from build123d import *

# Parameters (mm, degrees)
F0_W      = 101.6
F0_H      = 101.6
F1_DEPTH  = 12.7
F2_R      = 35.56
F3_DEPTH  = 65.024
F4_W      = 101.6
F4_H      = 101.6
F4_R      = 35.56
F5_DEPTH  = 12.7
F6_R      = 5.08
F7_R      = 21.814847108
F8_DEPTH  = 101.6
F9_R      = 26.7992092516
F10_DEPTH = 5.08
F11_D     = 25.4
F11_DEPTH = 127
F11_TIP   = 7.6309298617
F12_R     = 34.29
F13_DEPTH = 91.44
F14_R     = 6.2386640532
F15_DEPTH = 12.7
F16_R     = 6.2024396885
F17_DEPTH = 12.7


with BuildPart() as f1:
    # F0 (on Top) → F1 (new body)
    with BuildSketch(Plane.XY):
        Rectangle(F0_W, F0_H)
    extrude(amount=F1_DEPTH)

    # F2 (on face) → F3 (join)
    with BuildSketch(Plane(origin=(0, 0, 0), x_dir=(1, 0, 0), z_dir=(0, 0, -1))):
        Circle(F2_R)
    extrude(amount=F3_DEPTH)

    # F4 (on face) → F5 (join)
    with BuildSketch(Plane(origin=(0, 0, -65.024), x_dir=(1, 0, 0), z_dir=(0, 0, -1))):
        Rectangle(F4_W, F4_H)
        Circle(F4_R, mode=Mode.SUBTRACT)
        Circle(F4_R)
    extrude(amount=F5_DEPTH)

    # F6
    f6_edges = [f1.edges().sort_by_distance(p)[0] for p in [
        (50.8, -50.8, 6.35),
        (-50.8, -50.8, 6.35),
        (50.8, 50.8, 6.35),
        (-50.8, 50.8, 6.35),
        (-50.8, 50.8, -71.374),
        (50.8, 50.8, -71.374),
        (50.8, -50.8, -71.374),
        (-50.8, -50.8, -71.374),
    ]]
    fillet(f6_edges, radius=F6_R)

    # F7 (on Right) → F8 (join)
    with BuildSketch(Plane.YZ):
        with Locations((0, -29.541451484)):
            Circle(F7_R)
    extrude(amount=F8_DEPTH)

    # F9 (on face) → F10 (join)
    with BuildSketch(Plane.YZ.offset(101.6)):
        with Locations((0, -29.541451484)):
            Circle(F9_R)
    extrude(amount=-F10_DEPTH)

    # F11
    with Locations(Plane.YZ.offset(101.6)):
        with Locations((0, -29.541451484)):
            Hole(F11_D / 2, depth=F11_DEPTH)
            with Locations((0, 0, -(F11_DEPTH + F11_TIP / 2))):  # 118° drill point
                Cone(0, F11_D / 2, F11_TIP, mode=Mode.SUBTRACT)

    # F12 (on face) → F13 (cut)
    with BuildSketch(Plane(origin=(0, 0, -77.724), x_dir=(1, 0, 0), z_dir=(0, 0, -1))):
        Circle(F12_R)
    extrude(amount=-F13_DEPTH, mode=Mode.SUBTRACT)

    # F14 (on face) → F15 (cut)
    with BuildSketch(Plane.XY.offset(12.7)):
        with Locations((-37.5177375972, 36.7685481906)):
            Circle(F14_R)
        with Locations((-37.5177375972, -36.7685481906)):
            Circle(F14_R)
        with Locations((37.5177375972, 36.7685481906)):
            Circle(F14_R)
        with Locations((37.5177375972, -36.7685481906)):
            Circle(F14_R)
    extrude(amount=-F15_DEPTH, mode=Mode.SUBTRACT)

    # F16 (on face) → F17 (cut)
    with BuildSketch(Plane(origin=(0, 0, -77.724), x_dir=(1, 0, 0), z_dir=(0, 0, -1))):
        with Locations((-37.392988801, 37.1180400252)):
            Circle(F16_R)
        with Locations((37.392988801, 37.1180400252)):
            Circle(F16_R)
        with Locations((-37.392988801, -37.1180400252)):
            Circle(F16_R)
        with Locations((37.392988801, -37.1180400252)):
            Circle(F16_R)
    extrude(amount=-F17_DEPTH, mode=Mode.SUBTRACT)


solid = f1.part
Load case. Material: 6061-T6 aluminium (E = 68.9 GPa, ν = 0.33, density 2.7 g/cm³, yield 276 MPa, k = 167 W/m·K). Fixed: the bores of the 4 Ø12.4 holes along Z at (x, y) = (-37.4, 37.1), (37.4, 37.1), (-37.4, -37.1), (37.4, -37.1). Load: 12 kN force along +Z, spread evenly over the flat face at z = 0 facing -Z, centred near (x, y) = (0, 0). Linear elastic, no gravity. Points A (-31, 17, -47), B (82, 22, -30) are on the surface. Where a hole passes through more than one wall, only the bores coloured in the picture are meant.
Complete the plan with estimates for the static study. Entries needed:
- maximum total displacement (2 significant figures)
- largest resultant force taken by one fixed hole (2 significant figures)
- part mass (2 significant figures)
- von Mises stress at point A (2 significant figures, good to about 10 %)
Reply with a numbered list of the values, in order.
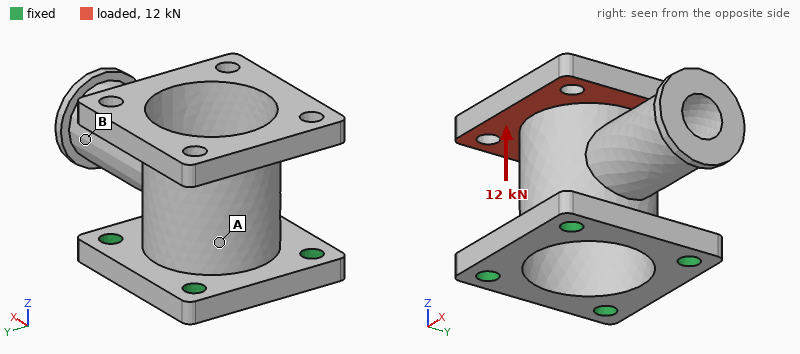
1. 0.19 mm
2. 3.0 kN
3. 660 g
4. 43 MPa
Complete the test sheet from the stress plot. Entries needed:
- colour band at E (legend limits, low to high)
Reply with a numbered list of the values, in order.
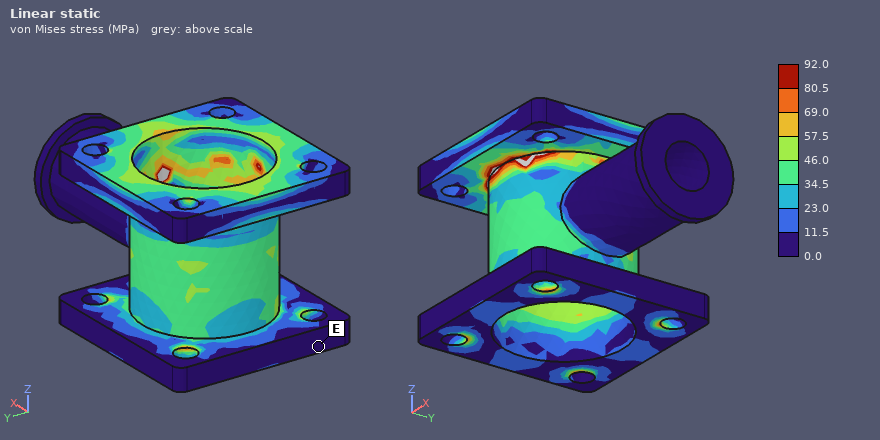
1. 0.0 to 11.5 MPa
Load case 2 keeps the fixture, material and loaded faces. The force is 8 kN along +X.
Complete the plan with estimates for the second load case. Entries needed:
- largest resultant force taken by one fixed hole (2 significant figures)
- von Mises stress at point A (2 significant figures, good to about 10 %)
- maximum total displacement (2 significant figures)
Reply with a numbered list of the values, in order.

1. 5.1 kN
2. 71 MPa
3. 0.40 mm
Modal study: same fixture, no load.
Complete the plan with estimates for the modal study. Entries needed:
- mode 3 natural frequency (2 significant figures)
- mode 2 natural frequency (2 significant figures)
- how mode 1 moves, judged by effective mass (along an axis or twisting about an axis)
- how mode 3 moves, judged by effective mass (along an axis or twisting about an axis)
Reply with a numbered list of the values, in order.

1. 1600 Hz
2. 1100 Hz
3. along Y
4. along Y
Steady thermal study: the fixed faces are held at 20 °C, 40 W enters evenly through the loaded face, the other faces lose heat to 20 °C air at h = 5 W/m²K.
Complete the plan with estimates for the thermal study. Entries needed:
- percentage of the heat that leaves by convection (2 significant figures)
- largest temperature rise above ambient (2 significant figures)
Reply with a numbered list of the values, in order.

1. 21 %
2. 45 K
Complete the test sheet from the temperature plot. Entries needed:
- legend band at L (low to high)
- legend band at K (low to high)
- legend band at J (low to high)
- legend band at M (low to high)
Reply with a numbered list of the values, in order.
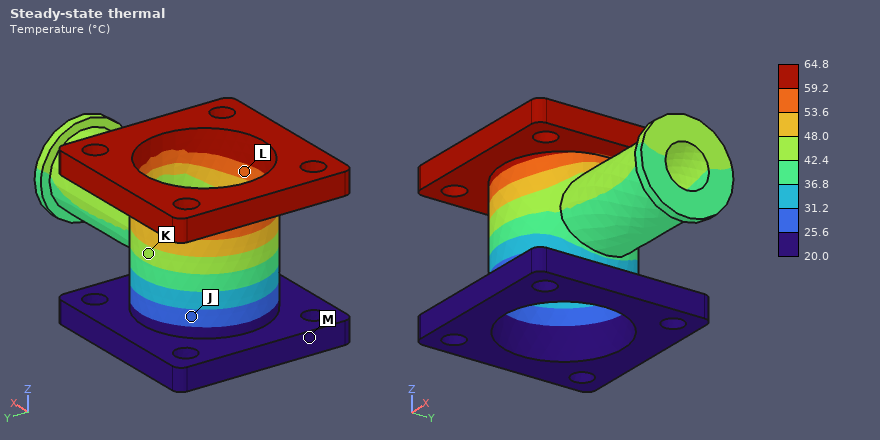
1. 53.6 to 59.2 °C
2. 42.4 to 48.0 °C
3. 25.6 to 31.2 °C
4. 20.0 to 25.6 °C
